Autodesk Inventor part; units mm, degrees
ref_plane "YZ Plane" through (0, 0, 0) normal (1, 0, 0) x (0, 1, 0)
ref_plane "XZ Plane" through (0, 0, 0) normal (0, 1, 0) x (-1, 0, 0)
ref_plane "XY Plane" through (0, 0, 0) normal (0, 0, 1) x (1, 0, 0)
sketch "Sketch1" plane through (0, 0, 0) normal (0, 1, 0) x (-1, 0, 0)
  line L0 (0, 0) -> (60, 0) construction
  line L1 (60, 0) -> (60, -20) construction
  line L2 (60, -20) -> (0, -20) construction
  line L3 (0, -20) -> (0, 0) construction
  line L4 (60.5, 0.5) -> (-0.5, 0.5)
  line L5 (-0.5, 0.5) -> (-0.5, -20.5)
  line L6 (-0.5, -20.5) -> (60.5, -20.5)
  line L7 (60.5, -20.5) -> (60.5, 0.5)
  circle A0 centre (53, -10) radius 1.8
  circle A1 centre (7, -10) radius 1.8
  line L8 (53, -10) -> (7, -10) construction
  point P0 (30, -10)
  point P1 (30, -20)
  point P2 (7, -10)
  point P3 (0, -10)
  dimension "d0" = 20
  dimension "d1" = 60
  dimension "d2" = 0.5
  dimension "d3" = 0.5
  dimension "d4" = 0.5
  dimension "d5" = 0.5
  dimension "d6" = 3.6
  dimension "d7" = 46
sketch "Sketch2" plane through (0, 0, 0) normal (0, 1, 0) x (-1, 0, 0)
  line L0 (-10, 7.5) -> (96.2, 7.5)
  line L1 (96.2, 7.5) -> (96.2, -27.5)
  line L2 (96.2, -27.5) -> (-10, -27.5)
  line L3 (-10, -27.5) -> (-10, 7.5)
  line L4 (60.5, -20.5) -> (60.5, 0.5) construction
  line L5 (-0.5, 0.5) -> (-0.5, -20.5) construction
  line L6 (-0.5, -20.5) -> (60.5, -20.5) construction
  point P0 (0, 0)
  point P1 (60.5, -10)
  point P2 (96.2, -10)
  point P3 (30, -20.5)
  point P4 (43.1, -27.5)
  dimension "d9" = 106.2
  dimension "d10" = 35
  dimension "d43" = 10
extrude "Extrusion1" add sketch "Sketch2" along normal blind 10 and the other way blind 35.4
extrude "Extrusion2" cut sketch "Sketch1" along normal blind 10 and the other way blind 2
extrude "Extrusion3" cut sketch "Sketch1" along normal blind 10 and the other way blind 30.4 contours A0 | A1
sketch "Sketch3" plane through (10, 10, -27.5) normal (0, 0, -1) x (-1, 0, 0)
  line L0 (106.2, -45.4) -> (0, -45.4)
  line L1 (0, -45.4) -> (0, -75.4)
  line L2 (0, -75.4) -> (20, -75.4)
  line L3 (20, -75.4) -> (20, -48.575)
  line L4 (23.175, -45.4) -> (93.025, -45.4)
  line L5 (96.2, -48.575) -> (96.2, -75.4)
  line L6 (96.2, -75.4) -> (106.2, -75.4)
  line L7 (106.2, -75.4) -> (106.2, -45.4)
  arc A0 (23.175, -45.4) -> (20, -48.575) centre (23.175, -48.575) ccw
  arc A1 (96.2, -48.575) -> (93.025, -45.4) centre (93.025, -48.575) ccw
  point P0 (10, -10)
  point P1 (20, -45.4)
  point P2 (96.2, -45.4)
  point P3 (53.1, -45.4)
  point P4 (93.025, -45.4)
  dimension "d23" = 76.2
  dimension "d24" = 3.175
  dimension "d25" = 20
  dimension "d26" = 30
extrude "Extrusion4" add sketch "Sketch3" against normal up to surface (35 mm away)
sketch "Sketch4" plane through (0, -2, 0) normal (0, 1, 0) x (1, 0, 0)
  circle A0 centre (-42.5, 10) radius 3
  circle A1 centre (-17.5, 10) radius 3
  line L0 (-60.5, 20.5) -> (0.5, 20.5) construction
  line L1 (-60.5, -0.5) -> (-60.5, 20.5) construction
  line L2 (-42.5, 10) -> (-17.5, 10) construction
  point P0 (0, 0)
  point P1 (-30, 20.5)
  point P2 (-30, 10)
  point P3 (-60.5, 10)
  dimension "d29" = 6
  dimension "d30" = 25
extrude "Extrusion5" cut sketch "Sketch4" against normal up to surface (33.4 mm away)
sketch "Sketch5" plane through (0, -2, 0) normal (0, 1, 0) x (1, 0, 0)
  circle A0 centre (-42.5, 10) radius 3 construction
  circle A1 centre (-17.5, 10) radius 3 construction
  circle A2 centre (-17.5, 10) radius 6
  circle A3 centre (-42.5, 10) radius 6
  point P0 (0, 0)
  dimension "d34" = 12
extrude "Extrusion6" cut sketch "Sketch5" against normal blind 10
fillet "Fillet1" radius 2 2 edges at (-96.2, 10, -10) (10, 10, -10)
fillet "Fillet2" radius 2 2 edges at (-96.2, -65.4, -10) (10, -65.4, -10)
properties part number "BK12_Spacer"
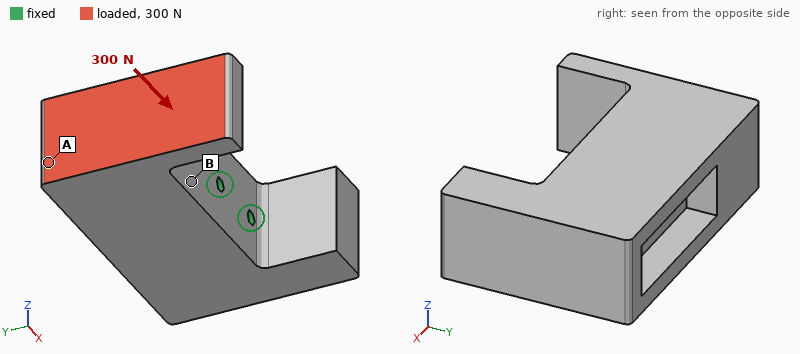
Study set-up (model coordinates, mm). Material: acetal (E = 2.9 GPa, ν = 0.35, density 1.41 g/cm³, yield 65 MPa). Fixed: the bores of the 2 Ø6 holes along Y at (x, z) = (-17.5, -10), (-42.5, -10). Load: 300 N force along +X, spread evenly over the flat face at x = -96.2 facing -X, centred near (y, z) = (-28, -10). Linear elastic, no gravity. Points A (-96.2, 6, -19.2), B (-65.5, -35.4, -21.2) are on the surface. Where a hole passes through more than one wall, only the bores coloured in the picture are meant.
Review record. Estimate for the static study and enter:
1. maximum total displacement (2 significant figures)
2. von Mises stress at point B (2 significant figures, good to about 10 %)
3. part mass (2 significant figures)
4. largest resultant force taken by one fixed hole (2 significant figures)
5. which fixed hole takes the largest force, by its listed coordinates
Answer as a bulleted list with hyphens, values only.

- 99 µm
- 0.61 MPa
- 250 g
- 240 N
- (-42.5, -10)
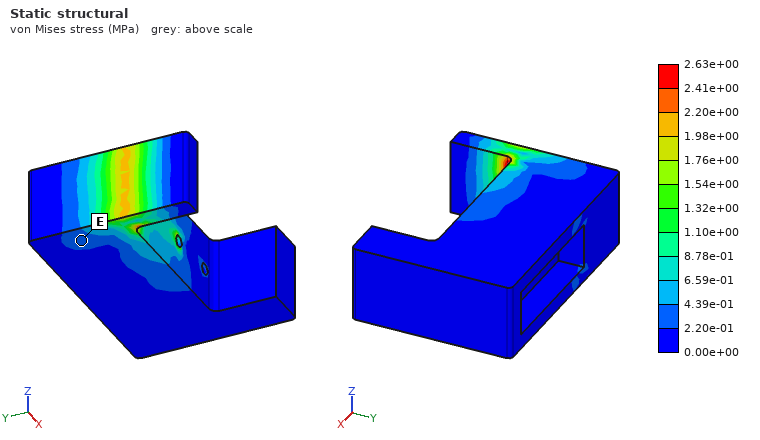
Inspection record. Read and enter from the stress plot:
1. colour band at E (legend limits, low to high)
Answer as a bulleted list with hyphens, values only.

- 2.20e-01 to 4.39e-01 MPa
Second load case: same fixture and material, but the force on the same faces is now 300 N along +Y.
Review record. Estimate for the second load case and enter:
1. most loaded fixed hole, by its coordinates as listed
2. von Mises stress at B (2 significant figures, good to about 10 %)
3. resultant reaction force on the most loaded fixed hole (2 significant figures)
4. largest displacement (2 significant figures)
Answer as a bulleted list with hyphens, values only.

- (-42.5, -10)
- 0.96 MPa
- 570 N
- 0.13 mm
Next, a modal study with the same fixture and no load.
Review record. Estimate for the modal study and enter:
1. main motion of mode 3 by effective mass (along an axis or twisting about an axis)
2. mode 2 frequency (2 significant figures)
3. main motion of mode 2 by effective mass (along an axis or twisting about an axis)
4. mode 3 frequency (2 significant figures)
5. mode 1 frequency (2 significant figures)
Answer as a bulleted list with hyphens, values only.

- twisting about X
- 1200 Hz
- along Y
- 1600 Hz
- 1200 Hz
